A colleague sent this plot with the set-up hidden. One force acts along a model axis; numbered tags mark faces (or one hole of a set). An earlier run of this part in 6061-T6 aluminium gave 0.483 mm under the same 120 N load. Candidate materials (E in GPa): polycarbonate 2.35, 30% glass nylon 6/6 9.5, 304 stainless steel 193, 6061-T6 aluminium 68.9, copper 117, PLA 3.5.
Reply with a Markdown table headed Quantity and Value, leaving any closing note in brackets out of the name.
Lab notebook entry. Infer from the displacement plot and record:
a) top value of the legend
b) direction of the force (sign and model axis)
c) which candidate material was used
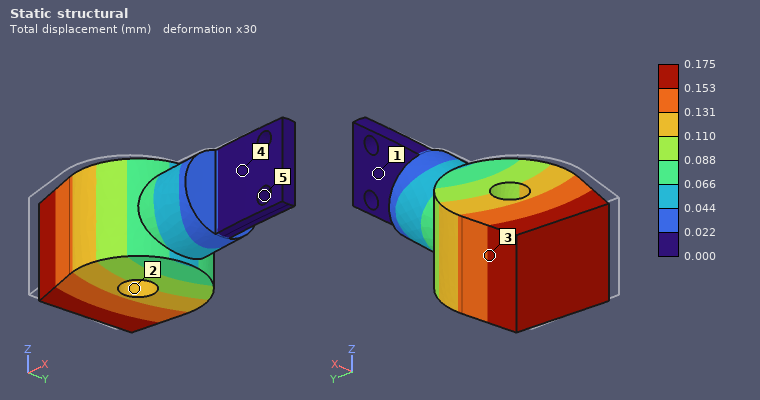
| Quantity | Value |
|---|---|
| top value of the legend | 0.175 mm |
| direction of the force | +Y |
| which candidate material was used | 304 stainless steel |
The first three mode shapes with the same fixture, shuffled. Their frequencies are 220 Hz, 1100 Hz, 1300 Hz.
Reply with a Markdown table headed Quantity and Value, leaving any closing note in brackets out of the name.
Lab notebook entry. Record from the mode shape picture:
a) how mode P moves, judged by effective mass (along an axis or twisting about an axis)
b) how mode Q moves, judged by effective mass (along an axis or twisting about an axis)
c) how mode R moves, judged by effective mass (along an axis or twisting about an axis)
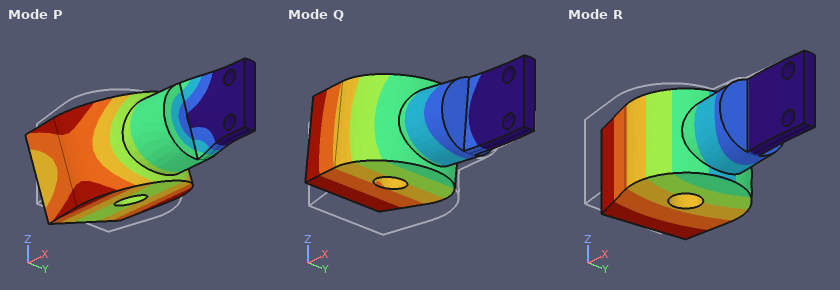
| Quantity | Value |
|---|---|
| how mode P moves, judged by effective mass | twisting about X |
| how mode Q moves, judged by effective mass | along Z |
| how mode R moves, judged by effective mass | along Y |
